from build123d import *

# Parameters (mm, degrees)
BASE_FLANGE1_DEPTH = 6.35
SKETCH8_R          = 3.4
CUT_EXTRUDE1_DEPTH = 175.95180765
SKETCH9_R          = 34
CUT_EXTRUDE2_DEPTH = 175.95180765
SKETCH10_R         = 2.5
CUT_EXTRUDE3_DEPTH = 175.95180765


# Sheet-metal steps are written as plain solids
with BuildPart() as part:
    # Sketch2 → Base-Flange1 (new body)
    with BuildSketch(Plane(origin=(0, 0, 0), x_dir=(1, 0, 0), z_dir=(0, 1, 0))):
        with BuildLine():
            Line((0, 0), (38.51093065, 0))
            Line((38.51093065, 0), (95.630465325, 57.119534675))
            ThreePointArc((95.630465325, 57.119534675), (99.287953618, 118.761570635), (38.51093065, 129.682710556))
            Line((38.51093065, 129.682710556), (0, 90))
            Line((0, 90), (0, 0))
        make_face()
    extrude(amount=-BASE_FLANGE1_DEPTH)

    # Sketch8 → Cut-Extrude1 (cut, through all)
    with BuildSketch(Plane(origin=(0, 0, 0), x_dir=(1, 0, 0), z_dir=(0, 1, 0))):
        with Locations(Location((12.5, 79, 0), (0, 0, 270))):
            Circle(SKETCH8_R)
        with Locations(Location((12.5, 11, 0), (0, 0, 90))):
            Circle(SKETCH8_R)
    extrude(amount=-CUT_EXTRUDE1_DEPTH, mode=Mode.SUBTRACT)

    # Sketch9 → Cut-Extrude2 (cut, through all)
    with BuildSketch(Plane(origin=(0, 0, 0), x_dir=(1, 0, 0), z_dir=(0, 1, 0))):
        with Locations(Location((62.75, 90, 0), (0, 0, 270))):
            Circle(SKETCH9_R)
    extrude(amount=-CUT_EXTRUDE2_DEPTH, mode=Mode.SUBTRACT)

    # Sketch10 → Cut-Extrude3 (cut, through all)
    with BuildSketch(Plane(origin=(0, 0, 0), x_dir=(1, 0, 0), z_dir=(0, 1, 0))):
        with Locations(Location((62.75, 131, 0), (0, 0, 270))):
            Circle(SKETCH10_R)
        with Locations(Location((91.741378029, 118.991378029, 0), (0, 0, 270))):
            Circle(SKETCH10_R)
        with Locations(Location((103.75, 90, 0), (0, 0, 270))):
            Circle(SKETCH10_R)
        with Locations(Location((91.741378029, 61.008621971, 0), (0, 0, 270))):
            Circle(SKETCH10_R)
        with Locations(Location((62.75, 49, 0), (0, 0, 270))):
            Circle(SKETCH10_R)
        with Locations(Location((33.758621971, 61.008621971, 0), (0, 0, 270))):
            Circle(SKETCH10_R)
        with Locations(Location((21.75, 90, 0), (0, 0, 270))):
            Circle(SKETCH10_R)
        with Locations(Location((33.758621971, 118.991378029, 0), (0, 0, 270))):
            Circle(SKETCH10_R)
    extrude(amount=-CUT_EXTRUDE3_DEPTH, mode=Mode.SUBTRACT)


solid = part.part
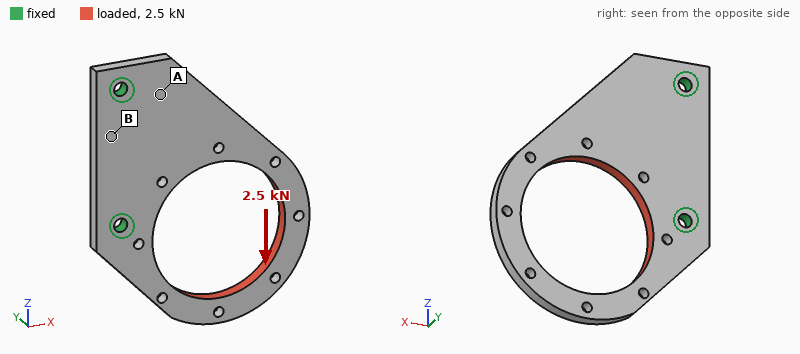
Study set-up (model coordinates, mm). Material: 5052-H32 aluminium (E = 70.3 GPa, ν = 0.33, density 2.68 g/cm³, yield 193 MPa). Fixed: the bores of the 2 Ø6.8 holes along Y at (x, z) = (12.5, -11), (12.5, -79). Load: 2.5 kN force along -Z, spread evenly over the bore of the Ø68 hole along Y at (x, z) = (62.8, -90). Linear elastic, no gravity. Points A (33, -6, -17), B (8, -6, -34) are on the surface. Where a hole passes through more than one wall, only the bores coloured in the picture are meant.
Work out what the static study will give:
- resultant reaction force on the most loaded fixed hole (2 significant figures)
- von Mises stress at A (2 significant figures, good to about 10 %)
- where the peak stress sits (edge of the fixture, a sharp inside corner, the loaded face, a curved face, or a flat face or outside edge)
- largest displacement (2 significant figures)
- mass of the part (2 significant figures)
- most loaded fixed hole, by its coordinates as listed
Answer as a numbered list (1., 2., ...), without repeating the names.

1. 2.3 kN
2. 13 MPa
3. a curved face
4. 0.14 mm
5. 120 g
6. (12.5, -79)
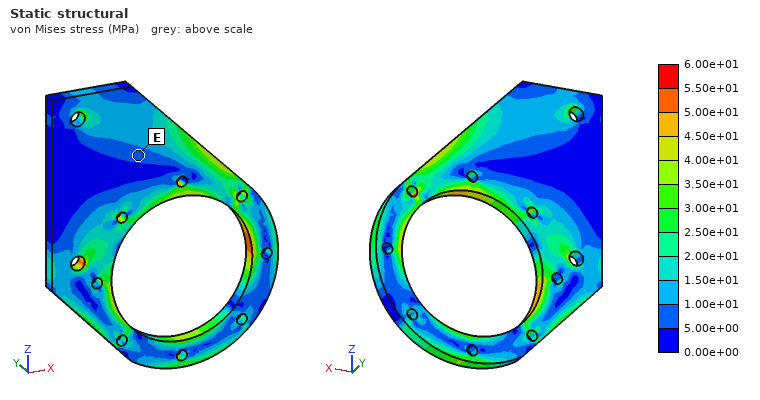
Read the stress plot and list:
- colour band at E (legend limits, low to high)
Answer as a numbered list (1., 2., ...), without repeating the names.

1. 5.00e+00 to 1.00e+01 MPa
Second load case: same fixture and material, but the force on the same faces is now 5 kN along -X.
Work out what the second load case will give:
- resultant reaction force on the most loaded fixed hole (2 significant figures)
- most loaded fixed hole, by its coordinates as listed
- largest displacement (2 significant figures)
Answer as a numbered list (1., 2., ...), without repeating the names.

1. 5.5 kN
2. (12.5, -79)
3. 0.28 mm
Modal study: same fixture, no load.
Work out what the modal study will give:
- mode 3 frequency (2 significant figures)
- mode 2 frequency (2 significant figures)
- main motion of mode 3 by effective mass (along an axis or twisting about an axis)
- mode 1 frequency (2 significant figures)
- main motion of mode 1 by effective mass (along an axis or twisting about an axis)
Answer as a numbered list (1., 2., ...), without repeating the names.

1. 2200 Hz
2. 1200 Hz
3. along Y
4. 540 Hz
5. along Y
